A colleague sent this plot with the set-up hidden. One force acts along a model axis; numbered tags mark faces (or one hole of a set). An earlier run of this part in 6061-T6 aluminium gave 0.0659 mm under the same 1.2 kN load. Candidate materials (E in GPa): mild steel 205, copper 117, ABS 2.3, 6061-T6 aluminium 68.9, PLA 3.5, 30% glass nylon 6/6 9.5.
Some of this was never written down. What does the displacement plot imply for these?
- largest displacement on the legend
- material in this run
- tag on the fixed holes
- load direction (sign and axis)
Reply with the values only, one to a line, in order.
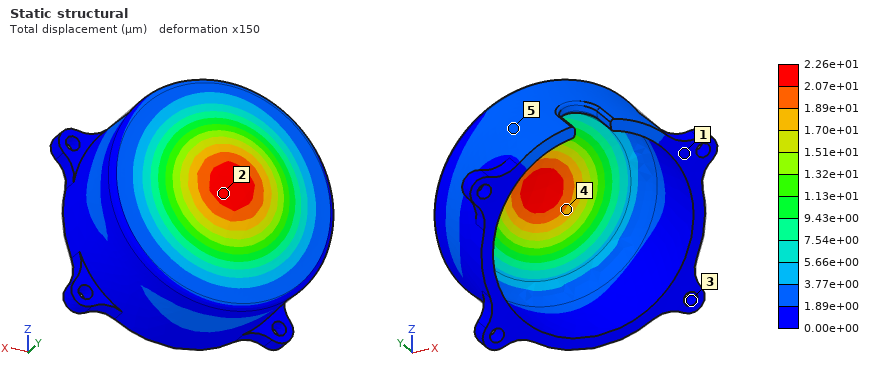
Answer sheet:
2.26e+01 µm
mild steel
3
+Y
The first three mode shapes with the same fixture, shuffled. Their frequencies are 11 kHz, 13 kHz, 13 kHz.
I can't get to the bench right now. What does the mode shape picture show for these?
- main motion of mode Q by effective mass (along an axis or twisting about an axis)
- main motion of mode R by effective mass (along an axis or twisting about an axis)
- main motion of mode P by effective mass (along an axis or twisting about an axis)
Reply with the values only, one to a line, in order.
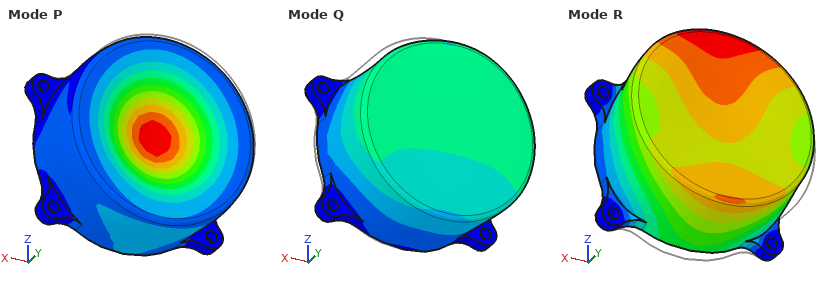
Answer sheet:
along X
along Z
along Y
